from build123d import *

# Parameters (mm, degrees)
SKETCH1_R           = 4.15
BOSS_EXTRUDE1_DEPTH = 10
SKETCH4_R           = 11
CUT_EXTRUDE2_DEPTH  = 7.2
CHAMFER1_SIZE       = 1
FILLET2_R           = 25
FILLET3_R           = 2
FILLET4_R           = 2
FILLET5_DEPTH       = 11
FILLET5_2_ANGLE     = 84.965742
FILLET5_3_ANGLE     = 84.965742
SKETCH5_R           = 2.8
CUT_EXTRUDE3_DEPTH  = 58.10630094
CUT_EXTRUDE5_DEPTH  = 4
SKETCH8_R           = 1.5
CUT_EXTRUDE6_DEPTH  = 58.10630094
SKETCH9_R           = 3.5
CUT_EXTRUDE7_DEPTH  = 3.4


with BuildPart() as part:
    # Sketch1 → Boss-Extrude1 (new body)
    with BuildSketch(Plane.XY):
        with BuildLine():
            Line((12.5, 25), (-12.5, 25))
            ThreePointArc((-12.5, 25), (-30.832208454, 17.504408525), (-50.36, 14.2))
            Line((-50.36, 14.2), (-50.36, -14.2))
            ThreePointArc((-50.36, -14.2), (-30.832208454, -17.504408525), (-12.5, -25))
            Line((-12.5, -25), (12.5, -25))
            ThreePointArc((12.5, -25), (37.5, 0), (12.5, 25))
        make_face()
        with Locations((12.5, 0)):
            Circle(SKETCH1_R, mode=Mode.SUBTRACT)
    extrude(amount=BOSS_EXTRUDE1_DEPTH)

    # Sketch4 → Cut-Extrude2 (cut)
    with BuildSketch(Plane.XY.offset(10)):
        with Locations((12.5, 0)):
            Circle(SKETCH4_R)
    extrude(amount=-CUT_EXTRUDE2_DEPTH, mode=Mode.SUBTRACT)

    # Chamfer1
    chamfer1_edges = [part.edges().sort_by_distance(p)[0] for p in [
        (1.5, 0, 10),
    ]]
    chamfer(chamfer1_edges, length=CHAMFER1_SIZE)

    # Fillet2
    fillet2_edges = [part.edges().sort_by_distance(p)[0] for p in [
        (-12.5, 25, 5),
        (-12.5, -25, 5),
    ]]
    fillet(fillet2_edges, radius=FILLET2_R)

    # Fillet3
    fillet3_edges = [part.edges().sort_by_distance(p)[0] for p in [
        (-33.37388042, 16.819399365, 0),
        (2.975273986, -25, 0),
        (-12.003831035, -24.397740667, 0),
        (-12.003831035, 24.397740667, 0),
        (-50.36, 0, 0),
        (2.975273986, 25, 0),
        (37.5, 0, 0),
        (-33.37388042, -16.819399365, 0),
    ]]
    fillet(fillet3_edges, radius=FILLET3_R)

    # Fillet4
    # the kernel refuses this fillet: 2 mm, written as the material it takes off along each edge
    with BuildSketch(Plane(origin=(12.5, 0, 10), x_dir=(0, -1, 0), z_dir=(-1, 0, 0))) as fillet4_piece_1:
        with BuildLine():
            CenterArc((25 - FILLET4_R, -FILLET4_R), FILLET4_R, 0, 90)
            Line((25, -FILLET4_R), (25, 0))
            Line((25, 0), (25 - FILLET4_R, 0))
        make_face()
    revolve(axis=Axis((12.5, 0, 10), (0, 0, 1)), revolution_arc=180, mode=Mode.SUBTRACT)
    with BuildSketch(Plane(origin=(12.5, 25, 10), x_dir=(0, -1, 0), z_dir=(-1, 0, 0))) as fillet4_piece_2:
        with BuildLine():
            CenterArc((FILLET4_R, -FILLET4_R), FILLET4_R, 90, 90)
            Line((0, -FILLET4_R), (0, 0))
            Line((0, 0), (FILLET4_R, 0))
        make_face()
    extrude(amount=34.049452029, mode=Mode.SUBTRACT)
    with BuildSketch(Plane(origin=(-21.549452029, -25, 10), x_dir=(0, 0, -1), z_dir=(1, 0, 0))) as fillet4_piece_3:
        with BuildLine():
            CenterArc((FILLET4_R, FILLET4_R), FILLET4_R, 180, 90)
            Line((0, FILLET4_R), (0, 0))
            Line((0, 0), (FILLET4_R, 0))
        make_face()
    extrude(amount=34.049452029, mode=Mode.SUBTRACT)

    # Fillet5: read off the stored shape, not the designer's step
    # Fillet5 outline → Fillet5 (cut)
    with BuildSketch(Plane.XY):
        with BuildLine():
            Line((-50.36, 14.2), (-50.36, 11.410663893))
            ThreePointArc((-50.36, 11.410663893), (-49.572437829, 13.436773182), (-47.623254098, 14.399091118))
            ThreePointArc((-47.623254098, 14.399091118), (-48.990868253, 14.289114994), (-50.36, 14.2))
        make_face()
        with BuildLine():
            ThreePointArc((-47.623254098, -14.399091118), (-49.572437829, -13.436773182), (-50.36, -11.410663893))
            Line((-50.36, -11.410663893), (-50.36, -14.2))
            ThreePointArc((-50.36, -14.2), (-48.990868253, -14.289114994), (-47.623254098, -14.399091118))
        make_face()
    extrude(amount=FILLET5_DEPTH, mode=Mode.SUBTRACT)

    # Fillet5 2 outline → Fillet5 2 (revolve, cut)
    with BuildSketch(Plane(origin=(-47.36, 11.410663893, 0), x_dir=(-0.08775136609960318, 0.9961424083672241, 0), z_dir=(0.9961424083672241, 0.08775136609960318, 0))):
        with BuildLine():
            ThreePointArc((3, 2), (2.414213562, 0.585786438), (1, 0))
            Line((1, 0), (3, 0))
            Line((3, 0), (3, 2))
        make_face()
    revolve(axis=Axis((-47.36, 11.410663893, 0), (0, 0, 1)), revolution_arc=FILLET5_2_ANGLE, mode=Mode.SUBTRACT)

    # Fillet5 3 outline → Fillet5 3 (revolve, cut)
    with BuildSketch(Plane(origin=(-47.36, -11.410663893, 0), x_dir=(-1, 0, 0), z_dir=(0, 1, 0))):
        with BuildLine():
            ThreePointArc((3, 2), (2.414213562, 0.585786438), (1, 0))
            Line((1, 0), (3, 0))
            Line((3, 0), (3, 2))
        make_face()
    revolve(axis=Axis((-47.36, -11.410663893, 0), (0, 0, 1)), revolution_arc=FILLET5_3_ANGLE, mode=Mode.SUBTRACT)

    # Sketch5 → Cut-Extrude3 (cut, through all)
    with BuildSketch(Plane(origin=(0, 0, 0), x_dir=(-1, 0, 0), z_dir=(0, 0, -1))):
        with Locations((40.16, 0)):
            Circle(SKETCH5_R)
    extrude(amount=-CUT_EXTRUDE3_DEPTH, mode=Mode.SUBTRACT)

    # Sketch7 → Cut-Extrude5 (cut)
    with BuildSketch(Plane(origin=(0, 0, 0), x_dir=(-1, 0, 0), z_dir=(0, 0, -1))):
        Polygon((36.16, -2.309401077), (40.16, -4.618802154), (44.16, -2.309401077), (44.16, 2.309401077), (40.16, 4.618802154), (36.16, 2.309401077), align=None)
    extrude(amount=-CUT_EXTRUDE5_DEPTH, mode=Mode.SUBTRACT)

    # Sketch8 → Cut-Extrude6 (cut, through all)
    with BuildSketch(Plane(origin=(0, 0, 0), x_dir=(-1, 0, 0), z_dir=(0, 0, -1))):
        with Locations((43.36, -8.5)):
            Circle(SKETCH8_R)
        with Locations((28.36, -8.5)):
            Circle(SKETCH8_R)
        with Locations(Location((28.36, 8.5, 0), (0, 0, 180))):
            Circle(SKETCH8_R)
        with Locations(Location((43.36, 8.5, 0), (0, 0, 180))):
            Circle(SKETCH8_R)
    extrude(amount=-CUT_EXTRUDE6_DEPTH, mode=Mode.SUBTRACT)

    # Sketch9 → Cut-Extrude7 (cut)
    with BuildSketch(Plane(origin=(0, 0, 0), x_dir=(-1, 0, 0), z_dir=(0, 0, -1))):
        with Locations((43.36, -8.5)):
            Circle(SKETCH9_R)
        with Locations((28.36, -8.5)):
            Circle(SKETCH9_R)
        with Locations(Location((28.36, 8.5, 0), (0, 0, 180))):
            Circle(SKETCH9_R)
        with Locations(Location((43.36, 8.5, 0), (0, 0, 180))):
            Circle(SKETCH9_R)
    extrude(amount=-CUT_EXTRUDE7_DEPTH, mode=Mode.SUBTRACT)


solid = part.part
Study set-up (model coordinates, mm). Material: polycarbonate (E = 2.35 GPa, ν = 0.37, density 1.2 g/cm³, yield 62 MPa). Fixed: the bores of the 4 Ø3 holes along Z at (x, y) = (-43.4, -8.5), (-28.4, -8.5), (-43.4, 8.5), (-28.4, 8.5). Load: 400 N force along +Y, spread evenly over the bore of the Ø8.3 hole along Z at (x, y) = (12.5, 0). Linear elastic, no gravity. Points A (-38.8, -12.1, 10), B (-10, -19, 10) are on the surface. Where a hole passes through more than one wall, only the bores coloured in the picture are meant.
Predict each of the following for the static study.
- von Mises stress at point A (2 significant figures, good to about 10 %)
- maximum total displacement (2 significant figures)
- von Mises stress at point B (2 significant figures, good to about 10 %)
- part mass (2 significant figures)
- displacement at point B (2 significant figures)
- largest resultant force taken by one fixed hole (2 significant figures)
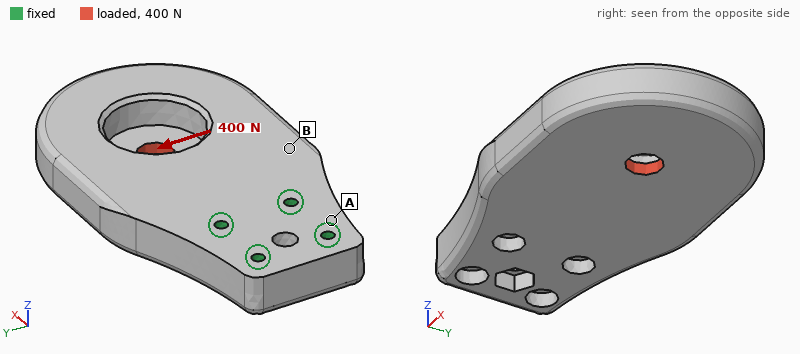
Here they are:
4.6 MPa
0.35 mm
1.9 MPa
38 g
0.12 mm
620 N
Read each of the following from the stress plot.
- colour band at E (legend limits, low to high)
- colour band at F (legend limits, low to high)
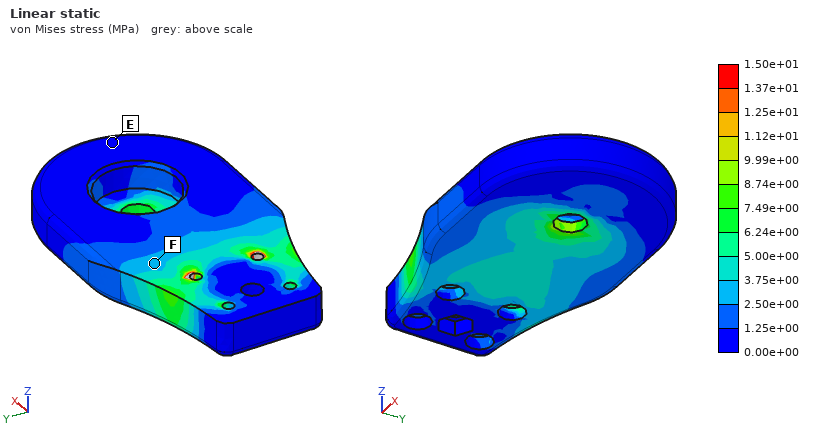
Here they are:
0.00e+00 to 1.25e+00 MPa
2.50e+00 to 3.75e+00 MPa
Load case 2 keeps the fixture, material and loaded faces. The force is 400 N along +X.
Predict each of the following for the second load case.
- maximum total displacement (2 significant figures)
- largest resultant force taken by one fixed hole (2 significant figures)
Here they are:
0.42 mm
140 N
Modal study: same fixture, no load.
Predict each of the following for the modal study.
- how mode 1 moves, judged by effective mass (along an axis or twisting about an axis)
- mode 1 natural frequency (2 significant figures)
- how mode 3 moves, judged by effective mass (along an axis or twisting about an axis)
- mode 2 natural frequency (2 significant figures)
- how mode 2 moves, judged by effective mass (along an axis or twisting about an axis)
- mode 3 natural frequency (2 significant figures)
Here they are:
along Z
490 Hz
along Y
1300 Hz
along Y
1400 Hz
